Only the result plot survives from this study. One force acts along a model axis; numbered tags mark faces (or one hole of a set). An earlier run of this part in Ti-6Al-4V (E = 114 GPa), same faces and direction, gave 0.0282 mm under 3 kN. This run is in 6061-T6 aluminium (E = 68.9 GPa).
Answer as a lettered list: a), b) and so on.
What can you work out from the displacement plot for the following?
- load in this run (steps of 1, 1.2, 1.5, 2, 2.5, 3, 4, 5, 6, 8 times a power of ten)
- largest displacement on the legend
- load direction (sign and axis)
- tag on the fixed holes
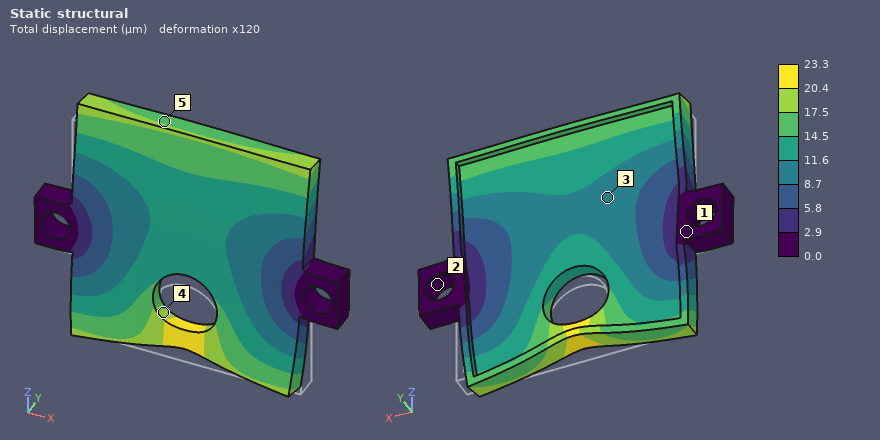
a) 1.5 kN
b) 23.3 µm
c) +Z
d) 2
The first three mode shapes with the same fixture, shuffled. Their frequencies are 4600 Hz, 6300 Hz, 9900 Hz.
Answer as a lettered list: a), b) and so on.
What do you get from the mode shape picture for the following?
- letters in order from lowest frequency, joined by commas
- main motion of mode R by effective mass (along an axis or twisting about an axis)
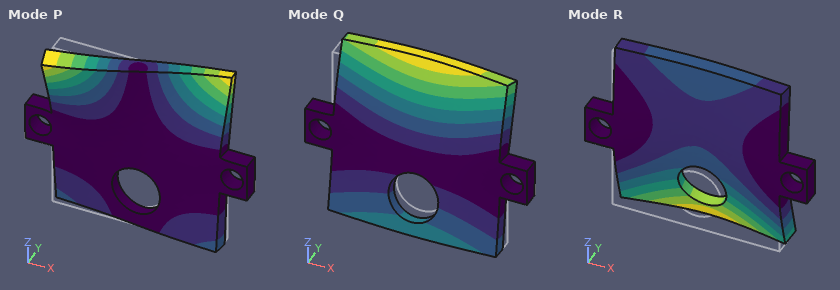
a) Q, R, P
b) along Y
